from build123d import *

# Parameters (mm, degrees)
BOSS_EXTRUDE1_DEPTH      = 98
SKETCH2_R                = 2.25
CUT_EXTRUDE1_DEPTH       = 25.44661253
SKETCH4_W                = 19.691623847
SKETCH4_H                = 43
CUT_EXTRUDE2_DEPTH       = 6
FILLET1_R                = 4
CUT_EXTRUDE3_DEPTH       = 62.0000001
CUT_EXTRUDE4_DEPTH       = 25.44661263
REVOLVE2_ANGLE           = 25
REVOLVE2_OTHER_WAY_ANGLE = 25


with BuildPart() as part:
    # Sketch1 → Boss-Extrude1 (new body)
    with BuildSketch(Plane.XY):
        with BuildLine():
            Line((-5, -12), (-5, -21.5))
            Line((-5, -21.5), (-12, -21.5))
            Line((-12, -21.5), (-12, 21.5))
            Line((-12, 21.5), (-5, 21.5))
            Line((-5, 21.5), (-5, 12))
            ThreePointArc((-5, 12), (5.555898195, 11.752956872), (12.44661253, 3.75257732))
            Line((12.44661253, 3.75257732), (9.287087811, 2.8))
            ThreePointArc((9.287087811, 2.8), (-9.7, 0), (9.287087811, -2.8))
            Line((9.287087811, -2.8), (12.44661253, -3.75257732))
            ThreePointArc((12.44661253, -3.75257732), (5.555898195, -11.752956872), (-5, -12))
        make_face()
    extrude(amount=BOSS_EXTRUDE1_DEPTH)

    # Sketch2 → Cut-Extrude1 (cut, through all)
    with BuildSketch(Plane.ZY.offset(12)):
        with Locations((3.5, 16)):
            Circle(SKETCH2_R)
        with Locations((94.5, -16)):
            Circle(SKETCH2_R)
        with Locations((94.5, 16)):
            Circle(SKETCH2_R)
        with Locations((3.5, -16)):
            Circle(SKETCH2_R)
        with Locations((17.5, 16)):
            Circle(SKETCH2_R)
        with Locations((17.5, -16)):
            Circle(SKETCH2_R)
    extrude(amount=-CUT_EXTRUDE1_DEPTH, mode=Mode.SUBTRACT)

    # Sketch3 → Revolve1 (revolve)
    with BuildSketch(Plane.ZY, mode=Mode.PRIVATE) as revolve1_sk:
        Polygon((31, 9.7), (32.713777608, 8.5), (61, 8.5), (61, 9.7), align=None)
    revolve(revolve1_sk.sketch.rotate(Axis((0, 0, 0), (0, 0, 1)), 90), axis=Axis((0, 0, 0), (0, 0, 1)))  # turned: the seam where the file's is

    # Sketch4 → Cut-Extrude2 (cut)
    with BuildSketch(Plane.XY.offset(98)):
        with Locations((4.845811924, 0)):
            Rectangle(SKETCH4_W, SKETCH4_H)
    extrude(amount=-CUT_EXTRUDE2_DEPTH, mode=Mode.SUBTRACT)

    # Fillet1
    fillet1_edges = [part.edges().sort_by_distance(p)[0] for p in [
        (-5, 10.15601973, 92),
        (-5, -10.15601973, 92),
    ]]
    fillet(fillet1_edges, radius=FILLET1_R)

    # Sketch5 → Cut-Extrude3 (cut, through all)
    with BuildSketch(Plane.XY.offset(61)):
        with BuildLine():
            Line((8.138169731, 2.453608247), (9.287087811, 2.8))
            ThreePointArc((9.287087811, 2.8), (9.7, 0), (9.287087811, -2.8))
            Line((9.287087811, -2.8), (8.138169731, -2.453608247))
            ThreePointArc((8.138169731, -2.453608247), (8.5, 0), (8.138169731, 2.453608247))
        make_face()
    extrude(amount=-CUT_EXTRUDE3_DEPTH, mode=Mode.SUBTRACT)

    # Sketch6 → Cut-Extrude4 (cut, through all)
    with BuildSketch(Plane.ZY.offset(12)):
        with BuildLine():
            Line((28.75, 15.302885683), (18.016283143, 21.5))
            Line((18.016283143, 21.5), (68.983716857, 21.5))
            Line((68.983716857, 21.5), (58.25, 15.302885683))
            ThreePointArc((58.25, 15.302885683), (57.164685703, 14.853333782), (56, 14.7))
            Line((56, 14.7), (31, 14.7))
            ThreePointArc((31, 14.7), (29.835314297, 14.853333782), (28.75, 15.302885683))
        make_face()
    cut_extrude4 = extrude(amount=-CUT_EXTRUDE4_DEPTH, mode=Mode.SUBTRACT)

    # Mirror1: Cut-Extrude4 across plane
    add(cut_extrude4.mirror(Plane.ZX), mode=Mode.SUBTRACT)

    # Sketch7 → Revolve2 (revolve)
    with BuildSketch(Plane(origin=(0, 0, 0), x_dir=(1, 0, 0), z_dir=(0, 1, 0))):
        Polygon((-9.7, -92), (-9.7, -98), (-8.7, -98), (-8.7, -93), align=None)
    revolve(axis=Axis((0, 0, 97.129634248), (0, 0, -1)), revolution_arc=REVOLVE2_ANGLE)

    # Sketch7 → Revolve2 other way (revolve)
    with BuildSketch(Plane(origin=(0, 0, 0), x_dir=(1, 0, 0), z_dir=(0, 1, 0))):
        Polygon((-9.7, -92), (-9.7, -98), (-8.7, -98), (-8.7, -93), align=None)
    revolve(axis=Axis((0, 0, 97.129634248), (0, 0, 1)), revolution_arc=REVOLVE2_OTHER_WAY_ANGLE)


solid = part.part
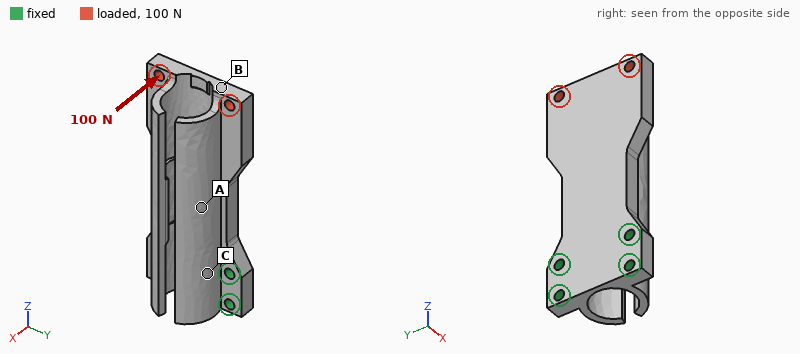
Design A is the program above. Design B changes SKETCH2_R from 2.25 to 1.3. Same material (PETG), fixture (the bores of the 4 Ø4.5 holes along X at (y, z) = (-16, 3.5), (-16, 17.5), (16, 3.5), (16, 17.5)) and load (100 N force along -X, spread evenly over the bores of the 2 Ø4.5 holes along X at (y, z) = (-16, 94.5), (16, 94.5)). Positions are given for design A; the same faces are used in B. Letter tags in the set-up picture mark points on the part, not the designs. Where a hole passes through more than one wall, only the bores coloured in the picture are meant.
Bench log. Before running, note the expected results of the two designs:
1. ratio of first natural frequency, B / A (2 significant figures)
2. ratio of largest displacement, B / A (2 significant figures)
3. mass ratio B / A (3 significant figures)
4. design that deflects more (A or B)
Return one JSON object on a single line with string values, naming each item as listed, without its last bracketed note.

{"ratio of first natural frequency, B / A": "0.92", "ratio of largest displacement, B / A": "1.1", "mass ratio B / A": "1.01", "design that deflects more": "B"}
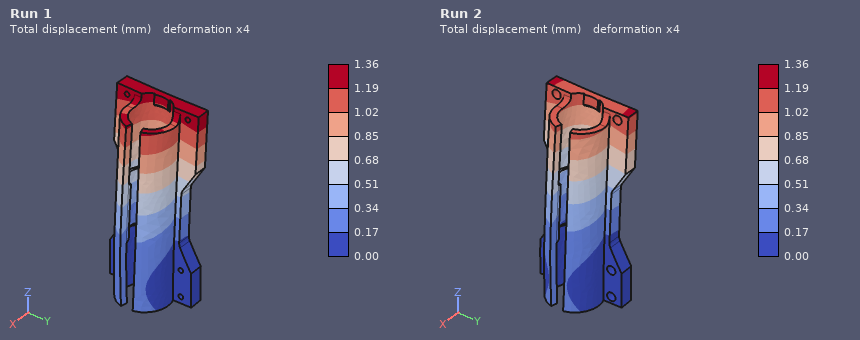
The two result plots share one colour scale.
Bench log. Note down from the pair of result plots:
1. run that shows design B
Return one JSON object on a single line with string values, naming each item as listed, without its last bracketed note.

{"run that shows design B": "Run 1"}
